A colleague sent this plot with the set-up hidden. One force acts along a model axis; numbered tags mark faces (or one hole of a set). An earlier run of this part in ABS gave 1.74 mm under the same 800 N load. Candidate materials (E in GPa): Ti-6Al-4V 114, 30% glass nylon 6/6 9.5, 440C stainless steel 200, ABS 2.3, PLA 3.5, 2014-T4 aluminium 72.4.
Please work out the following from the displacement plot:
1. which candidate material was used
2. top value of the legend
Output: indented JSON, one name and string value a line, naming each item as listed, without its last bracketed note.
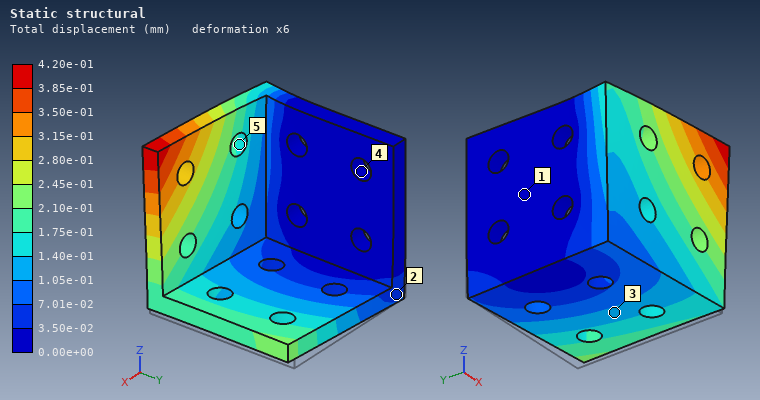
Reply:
{
  "which candidate material was used": "30% glass nylon 6/6",
  "top value of the legend": "4.20e-01 mm"
}
